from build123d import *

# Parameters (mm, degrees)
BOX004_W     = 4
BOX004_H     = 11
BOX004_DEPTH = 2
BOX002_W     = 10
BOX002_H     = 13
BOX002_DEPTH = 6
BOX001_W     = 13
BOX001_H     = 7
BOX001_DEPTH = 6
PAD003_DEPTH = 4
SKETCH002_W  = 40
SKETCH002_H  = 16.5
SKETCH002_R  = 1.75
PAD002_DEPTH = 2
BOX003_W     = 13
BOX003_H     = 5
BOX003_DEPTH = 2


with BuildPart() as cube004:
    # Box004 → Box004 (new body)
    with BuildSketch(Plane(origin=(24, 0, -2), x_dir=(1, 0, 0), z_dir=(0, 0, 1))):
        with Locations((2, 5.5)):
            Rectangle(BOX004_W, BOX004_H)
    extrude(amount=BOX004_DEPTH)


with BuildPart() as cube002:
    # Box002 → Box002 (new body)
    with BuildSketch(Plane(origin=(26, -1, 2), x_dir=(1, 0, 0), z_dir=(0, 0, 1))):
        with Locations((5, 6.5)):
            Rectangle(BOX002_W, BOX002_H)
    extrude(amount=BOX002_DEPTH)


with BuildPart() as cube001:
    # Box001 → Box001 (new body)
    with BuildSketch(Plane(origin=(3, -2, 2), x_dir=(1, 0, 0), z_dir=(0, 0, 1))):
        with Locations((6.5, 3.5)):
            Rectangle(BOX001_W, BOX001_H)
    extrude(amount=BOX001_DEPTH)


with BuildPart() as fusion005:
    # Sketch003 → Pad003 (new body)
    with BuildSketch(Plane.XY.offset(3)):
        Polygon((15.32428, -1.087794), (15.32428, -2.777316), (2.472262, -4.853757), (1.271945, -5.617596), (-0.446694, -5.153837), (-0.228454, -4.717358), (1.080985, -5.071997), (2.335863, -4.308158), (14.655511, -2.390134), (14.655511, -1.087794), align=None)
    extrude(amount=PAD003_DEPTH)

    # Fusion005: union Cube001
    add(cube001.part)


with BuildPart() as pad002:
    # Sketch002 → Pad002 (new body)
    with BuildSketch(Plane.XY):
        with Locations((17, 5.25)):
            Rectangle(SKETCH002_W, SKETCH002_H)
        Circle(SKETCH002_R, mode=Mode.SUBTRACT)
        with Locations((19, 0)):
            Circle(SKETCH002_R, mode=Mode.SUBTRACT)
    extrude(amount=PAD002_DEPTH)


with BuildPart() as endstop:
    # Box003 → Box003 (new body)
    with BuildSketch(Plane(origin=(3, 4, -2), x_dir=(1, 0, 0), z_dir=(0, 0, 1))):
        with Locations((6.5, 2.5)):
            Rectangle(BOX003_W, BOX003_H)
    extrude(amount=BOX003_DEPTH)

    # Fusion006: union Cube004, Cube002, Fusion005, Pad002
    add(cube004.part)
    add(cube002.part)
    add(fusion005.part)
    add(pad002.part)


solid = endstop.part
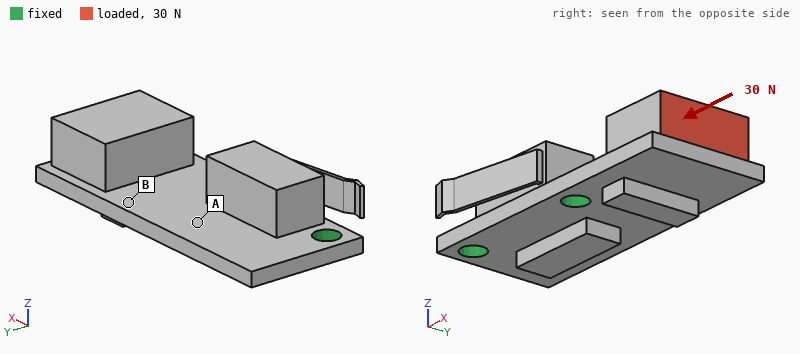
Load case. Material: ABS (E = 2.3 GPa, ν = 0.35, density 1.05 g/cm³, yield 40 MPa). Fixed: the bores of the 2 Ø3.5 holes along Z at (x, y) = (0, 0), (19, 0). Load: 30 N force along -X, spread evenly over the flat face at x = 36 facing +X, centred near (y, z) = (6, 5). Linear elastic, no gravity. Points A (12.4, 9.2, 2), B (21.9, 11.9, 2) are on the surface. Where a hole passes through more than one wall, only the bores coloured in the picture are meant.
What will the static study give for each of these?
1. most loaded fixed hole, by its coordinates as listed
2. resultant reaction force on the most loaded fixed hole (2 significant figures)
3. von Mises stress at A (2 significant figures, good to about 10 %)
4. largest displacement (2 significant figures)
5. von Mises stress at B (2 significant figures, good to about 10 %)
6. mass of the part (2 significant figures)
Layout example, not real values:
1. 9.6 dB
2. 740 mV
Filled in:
1. (19, 0)
2. 22 N
3. 1.7 MPa
4. 0.52 mm
5. 8.0 MPa
6. 3.0 g
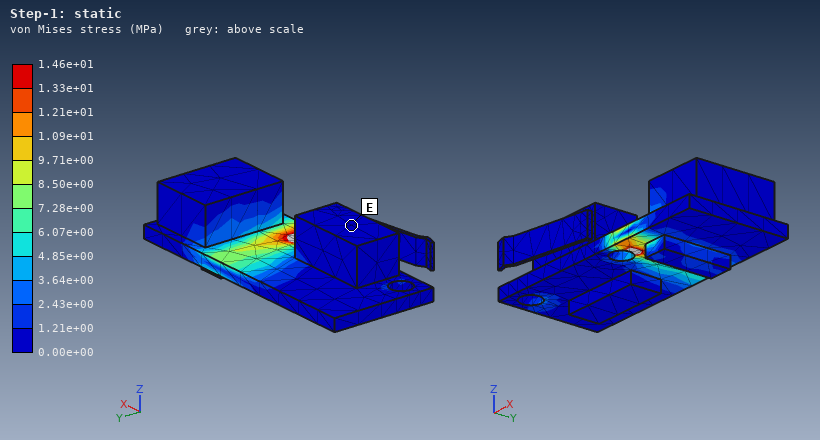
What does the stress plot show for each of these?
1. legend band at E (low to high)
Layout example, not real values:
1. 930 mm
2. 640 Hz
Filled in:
1. 0.00e+00 to 1.21e+00 MPa
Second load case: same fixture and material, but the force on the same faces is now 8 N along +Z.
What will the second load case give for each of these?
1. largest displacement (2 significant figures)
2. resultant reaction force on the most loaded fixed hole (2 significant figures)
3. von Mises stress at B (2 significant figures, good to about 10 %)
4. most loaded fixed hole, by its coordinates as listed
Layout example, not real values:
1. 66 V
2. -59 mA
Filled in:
1. 0.52 mm
2. 10 N
3. 6.0 MPa
4. (19, 0)
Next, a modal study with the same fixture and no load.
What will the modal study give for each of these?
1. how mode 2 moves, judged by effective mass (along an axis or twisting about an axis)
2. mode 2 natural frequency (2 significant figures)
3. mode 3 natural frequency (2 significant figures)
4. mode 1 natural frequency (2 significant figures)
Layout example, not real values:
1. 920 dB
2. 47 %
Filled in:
1. along Z
2. 820 Hz
3. 2100 Hz
4. 480 Hz
